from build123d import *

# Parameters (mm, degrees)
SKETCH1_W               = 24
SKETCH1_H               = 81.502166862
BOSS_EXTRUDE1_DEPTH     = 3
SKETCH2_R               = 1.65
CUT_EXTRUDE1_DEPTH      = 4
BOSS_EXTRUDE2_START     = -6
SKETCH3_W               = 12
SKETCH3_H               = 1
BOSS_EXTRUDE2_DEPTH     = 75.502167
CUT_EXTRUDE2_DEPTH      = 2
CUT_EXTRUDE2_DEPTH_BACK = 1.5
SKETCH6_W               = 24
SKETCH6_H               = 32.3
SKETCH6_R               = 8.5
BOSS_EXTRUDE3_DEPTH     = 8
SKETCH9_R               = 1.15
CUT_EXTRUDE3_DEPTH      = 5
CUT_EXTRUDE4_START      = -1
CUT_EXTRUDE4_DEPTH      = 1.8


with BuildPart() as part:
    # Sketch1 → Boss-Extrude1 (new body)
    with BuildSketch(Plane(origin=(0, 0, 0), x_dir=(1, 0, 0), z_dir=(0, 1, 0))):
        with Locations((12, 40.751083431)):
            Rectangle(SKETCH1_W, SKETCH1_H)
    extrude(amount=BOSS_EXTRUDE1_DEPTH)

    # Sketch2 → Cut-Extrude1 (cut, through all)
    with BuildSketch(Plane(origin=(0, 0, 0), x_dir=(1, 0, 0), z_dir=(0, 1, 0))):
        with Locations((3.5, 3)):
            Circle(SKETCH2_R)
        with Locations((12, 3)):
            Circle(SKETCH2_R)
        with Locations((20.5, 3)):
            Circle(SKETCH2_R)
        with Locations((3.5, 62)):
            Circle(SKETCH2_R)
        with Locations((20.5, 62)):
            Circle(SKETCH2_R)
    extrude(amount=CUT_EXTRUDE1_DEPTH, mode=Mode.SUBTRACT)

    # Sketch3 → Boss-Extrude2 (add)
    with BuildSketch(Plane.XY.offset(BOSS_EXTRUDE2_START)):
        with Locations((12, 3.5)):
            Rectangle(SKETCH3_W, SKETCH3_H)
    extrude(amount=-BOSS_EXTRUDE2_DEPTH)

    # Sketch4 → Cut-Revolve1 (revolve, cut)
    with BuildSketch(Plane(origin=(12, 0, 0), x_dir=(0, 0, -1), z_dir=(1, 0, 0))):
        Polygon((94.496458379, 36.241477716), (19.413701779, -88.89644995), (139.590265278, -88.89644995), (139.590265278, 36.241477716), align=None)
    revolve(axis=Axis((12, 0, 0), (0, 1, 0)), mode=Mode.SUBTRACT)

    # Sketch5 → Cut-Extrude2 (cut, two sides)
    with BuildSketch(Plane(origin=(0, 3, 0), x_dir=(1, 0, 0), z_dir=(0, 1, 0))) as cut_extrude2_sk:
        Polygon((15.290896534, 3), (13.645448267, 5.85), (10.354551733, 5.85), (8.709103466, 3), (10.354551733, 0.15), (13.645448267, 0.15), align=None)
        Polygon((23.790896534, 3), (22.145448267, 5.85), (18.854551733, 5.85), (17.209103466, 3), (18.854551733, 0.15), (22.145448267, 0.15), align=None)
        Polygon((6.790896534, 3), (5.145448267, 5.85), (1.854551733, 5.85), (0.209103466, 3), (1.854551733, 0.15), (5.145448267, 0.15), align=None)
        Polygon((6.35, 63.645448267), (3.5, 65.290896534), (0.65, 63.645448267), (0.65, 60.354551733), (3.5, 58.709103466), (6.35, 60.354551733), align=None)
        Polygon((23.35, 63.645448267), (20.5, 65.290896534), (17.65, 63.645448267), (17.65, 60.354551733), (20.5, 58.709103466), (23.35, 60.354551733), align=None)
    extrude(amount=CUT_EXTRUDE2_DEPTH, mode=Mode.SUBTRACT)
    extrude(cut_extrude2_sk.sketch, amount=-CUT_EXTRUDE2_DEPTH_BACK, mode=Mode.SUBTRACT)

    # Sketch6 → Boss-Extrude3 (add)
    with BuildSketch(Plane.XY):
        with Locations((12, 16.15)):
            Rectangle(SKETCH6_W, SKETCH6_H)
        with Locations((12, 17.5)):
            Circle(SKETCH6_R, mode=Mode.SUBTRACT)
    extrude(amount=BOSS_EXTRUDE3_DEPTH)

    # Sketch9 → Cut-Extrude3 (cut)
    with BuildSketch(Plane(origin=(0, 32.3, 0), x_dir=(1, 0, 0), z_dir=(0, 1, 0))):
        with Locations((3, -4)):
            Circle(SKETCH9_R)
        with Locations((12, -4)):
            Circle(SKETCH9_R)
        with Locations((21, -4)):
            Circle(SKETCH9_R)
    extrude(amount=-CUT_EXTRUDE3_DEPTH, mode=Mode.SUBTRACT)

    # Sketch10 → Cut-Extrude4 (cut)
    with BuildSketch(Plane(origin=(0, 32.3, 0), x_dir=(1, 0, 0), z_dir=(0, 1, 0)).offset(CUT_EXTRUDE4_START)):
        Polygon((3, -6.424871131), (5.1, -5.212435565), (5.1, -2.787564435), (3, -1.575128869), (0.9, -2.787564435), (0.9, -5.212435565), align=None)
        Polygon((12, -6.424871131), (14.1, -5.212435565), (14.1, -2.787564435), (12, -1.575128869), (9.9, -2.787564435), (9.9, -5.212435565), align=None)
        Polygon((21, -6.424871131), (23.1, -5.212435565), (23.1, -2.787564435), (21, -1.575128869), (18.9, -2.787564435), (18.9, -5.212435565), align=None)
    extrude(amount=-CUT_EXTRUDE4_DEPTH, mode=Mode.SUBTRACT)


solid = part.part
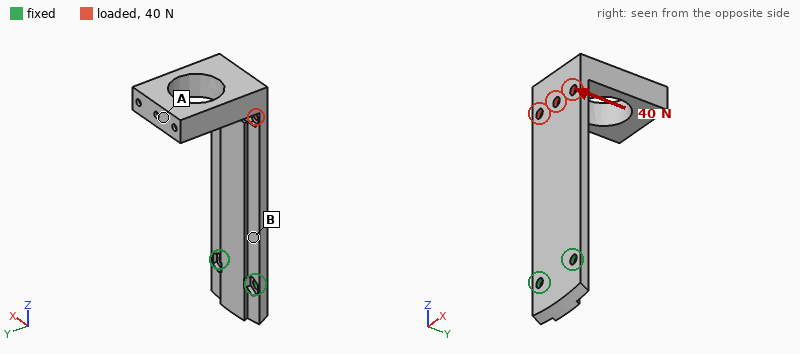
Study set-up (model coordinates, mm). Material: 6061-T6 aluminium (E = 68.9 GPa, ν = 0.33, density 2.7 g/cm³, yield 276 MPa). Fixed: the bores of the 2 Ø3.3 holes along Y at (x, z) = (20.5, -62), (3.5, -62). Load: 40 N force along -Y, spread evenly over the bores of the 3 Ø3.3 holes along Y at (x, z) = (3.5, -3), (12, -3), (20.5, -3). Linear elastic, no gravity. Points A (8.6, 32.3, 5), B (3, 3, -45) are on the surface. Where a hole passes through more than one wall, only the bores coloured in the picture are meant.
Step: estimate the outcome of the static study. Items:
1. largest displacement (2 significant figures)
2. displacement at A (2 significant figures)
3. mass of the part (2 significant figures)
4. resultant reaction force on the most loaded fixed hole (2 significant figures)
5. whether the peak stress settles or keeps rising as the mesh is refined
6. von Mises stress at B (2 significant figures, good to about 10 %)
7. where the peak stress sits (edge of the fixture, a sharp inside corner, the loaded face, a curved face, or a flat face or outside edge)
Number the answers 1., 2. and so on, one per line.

1. 0.83 mm
2. 0.80 mm
3. 27 g
4. 75 N
5. keeps rising
6. 22 MPa
7. edge of the fixture
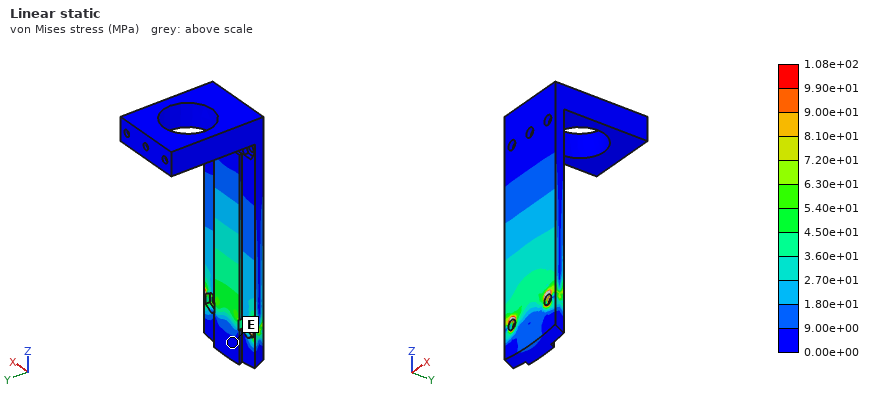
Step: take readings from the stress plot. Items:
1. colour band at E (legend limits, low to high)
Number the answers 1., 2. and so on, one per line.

1. 0.00e+00 to 9.00e+00 MPa
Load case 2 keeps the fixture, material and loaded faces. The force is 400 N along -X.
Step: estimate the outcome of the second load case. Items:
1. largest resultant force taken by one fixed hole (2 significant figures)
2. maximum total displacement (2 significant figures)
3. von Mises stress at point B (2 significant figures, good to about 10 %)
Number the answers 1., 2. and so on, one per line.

1. 1.3 kN
2. 0.20 mm
3. 40 MPa
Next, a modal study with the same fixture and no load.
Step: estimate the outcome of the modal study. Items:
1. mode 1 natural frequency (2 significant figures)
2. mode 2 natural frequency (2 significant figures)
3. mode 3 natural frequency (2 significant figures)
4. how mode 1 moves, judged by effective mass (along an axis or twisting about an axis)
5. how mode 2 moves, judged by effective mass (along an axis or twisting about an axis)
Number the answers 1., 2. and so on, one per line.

1. 290 Hz
2. 880 Hz
3. 1200 Hz
4. along Y
5. along X
